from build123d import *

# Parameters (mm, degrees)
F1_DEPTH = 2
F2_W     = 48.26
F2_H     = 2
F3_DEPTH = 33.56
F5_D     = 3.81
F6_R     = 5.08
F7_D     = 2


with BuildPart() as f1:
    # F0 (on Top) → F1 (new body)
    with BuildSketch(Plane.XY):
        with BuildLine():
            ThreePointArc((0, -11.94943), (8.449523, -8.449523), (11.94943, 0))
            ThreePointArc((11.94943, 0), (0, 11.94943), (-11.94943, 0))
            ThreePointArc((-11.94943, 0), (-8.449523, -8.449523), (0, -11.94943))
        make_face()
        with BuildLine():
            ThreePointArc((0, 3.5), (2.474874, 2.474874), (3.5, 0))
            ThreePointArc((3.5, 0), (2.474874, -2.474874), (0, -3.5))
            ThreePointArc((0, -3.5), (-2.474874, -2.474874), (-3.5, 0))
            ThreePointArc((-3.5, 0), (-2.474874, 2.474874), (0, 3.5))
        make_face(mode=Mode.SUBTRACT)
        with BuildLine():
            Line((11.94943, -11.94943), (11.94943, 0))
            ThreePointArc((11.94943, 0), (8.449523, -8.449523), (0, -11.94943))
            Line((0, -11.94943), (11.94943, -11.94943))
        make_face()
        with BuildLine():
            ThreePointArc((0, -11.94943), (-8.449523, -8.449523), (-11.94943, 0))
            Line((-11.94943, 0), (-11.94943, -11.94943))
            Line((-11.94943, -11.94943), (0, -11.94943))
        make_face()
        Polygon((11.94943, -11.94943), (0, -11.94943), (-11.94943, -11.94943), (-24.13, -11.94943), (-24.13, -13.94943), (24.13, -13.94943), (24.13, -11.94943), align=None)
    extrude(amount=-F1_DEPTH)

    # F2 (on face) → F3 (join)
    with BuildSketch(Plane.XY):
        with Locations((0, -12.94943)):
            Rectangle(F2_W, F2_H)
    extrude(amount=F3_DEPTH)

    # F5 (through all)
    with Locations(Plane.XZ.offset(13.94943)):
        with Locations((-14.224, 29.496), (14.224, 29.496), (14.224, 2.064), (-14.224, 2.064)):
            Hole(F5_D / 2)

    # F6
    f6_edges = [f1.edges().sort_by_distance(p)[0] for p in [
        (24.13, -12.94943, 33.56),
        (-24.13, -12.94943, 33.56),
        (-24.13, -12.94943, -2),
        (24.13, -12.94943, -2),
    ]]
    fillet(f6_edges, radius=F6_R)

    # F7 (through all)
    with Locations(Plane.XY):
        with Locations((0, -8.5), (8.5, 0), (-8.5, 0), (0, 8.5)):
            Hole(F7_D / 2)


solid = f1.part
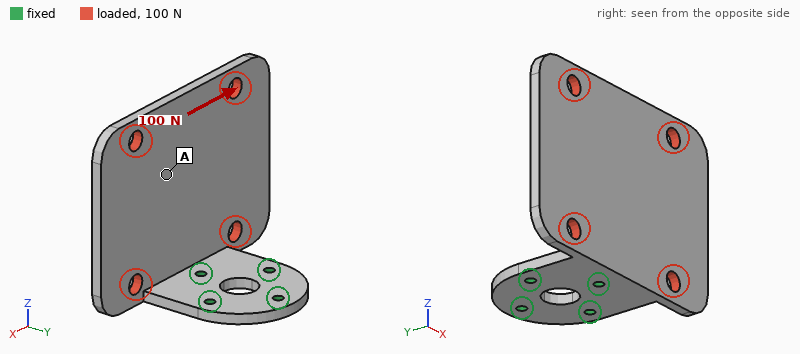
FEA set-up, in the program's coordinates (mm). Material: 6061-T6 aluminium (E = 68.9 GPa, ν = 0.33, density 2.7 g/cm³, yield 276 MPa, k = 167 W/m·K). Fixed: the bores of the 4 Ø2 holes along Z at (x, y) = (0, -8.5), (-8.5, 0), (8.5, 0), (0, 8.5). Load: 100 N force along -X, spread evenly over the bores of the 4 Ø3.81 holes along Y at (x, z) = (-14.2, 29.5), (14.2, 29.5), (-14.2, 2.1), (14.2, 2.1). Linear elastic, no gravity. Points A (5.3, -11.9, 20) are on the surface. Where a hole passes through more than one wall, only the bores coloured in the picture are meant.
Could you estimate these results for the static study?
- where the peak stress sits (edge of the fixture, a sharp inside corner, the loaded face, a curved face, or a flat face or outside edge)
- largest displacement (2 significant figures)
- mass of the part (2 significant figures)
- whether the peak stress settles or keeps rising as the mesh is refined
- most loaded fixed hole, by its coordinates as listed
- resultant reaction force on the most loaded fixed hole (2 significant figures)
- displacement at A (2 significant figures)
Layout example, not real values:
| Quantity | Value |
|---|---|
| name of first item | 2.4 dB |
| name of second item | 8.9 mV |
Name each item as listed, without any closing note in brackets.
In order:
| Quantity | Value |
|---|---|
| where the peak stress sits | edge of the fixture |
| largest displacement | 0.16 mm |
| mass of the part | 11 g |
| whether the peak stress settles or keeps rising as the mesh is refined | keeps rising |
| most loaded fixed hole, by its coordinates as listed | (0, -8.5) |
| resultant reaction force on the most loaded fixed hole | 88 N |
| displacement at A | 0.085 mm |
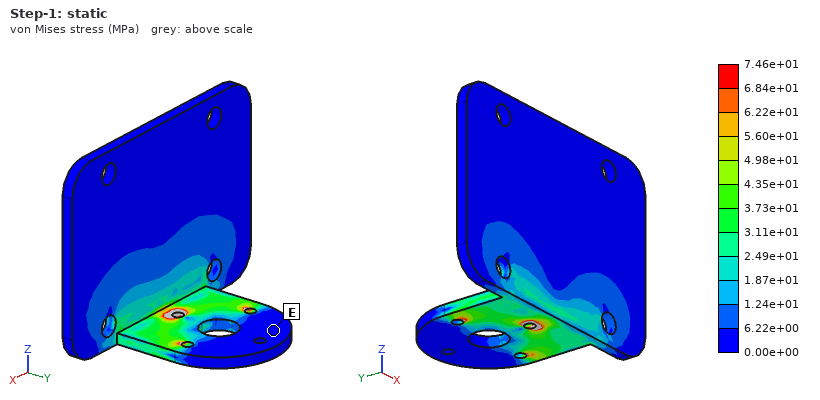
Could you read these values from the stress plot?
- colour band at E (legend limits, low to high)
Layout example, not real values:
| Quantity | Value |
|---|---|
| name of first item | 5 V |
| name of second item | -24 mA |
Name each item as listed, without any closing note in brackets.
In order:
| Quantity | Value |
|---|---|
| colour band at E | 0.00e+00 to 6.22e+00 MPa |
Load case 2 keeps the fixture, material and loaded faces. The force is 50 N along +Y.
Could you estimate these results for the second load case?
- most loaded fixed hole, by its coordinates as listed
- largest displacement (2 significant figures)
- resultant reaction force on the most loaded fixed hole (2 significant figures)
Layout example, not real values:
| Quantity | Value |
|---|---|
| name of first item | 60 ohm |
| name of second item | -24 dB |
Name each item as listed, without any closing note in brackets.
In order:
| Quantity | Value |
|---|---|
| most loaded fixed hole, by its coordinates as listed | (0, -8.5) |
| largest displacement | 0.28 mm |
| resultant reaction force on the most loaded fixed hole | 67 N |
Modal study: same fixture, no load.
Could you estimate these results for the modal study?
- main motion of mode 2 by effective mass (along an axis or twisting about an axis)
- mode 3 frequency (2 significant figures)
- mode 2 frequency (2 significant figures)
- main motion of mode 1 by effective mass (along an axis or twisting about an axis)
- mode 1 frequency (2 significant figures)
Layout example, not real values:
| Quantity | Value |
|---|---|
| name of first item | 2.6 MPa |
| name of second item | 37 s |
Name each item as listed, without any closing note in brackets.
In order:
| Quantity | Value |
|---|---|
| main motion of mode 2 by effective mass | along X |
| mode 3 frequency | 2000 Hz |
| mode 2 frequency | 1400 Hz |
| main motion of mode 1 by effective mass | along Y |
| mode 1 frequency | 920 Hz |
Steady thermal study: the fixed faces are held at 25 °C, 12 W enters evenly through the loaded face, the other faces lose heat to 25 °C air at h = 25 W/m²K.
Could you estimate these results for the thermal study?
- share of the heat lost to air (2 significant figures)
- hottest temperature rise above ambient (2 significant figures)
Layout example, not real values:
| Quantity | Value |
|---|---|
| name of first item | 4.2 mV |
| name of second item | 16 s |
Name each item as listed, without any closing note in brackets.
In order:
| Quantity | Value |
|---|---|
| share of the heat lost to air | 15 % |
| hottest temperature rise above ambient | 27 K |
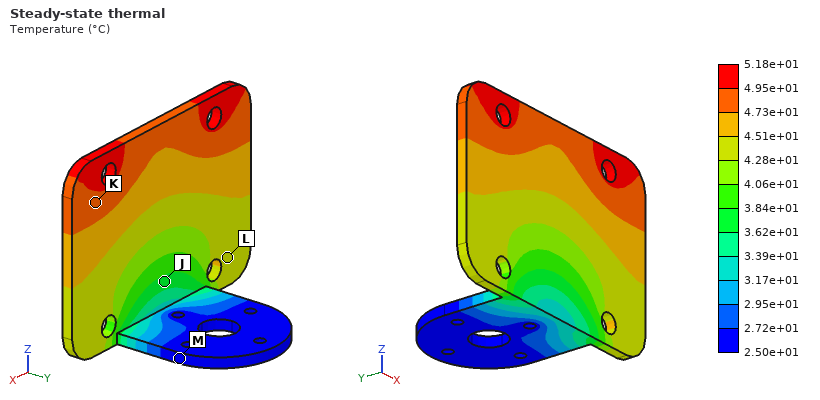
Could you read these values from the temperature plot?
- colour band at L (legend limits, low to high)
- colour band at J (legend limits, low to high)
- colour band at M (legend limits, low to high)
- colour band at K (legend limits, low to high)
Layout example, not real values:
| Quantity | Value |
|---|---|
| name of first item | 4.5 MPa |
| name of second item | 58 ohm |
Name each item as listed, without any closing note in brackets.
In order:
| Quantity | Value |
|---|---|
| colour band at L | 4.28e+01 to 4.51e+01 °C |
| colour band at J | 3.62e+01 to 3.84e+01 °C |
| colour band at M | 2.50e+01 to 2.72e+01 °C |
| colour band at K | 4.73e+01 to 4.95e+01 °C |
